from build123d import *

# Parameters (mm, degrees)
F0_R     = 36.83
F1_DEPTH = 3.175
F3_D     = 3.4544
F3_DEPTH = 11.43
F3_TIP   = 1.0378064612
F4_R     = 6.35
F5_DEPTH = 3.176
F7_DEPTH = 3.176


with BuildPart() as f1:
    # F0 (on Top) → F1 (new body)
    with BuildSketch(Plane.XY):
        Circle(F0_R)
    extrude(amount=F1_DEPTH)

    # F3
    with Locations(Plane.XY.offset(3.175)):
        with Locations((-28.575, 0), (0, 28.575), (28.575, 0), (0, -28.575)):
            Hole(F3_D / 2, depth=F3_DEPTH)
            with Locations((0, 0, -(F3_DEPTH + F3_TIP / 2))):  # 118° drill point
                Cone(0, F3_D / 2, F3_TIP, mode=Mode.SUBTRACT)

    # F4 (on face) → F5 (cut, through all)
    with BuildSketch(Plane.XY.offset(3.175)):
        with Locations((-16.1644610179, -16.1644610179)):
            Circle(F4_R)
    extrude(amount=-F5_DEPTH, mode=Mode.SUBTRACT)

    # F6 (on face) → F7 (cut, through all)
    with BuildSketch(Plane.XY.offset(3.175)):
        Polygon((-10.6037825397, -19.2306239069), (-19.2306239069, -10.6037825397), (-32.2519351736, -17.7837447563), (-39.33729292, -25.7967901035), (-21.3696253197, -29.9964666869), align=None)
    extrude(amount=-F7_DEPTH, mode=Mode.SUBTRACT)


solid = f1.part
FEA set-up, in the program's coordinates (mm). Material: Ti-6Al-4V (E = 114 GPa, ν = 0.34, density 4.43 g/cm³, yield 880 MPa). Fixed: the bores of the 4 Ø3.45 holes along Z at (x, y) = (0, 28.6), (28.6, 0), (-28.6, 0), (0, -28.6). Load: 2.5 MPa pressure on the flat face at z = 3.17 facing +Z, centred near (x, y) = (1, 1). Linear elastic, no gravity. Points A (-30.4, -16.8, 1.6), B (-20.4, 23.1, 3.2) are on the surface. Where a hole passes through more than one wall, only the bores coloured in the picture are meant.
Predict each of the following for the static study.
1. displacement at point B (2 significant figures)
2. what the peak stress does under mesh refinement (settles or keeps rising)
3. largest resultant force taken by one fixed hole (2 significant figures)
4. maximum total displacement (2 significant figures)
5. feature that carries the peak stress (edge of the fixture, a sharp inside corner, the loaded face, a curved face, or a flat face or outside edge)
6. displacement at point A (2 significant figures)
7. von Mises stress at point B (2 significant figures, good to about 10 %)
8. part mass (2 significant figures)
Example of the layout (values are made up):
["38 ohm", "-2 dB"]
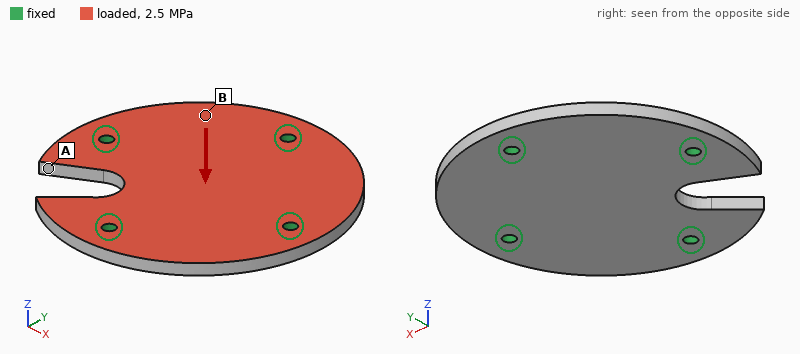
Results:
["0.098 mm", "keeps rising", "2.7 kN", "0.12 mm", "edge of the fixture", "0.028 mm", "110 MPa", "56 g"]
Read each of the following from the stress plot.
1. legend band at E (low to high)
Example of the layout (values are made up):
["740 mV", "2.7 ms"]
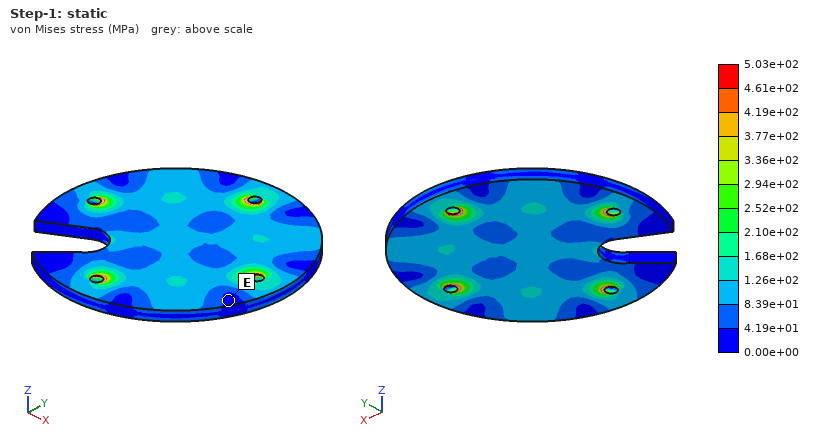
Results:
["0.00e+00 to 4.19e+01 MPa"]
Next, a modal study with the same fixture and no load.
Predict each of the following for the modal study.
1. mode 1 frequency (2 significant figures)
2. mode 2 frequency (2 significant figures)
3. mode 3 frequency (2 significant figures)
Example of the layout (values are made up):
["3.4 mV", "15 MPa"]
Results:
["6800 Hz", "7200 Hz", "7200 Hz"]
